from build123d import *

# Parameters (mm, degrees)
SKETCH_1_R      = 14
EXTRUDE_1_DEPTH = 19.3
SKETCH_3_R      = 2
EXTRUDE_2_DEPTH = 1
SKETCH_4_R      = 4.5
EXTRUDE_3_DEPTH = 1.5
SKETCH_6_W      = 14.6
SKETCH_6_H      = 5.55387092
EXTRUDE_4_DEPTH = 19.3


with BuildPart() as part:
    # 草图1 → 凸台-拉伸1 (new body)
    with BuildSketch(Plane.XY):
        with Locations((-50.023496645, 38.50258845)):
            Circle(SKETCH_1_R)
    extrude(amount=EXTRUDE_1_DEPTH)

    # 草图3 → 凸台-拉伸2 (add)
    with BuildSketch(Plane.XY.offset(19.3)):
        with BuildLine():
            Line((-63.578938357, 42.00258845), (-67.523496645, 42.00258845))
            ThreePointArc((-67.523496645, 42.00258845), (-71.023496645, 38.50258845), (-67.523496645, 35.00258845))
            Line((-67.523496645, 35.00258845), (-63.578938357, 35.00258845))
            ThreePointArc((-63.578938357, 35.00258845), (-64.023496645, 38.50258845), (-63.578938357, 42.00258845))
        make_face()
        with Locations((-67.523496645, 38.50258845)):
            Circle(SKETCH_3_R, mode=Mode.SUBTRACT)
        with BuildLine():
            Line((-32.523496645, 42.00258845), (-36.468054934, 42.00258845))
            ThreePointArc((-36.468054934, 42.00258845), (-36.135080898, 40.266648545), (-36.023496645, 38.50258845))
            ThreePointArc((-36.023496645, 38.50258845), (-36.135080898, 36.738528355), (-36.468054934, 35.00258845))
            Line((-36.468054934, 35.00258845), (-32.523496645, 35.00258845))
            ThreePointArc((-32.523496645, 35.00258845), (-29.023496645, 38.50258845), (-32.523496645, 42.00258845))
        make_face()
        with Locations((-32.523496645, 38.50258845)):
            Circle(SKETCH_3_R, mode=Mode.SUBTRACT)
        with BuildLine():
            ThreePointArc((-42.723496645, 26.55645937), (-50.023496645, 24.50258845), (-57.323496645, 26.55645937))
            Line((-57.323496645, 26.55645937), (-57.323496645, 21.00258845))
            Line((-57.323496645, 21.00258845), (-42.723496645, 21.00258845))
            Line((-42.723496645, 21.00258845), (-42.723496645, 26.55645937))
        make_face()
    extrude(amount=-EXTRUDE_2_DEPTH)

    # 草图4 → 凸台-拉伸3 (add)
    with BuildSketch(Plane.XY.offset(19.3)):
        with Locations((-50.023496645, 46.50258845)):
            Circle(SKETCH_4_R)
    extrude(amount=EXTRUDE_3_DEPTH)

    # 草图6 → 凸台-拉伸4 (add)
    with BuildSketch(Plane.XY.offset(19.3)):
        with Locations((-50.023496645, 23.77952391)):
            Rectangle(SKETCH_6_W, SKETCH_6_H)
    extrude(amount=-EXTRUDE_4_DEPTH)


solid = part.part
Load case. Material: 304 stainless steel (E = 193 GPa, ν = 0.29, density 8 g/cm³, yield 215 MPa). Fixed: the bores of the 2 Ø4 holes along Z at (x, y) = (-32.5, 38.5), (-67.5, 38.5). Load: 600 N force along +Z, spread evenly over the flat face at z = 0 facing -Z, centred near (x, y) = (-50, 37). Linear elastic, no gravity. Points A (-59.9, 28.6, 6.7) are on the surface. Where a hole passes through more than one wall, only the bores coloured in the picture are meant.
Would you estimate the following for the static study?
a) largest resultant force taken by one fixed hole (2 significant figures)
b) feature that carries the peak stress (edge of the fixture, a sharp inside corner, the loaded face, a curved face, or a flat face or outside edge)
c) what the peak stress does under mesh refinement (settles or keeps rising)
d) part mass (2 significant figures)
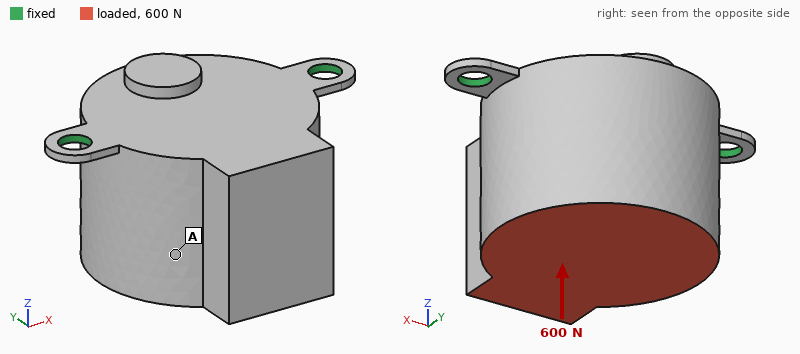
350 N
edge of the fixture
keeps rising
110 g
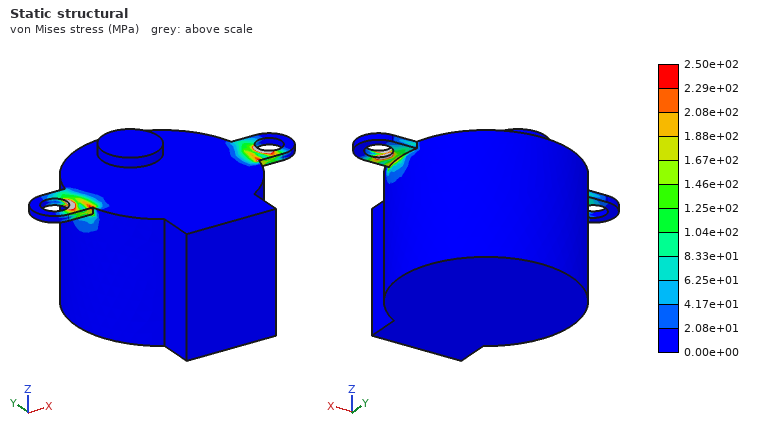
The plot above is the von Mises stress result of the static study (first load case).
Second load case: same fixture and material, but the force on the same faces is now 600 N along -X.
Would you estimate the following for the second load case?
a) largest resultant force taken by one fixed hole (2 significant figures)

490 N
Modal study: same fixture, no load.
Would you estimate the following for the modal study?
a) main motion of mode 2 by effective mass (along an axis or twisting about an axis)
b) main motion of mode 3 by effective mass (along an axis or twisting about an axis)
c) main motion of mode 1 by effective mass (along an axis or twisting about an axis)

along Z
along X
along Y
